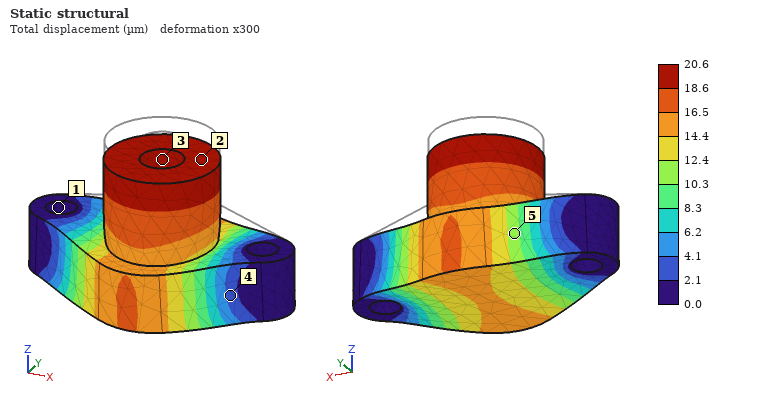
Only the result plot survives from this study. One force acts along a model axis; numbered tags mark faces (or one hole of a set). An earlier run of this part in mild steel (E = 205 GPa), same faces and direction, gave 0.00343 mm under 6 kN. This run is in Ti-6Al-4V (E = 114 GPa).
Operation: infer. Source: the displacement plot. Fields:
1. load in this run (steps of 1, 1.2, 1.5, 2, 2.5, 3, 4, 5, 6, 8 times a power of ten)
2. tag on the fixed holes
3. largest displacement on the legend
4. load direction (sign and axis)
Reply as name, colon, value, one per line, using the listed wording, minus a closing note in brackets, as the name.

load in this run: 20 kN
tag on the fixed holes: 1
largest displacement on the legend: 20.6 µm
load direction: -Z
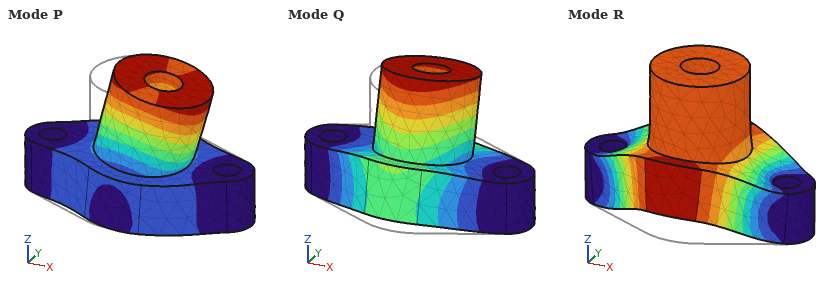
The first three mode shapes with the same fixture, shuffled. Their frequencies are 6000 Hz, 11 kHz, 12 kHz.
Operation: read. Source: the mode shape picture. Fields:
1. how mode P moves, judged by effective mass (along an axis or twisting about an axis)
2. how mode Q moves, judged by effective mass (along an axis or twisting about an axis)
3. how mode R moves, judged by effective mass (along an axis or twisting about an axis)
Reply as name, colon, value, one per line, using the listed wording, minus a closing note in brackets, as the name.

how mode P moves, judged by effective mass: along X
how mode Q moves, judged by effective mass: along Y
how mode R moves, judged by effective mass: along Z
